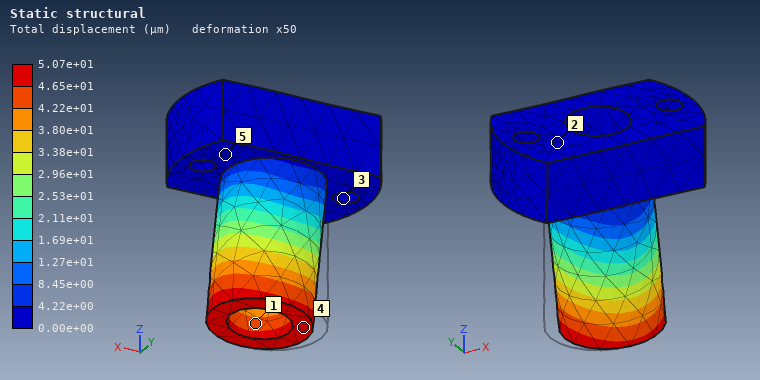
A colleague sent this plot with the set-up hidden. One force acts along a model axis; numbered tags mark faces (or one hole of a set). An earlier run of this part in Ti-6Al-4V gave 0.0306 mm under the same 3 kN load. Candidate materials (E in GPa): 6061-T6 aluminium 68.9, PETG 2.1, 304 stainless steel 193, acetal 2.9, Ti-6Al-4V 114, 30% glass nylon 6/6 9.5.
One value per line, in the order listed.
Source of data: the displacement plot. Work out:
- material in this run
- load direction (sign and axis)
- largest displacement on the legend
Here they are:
6061-T6 aluminium
+X
5.07e+01 µm
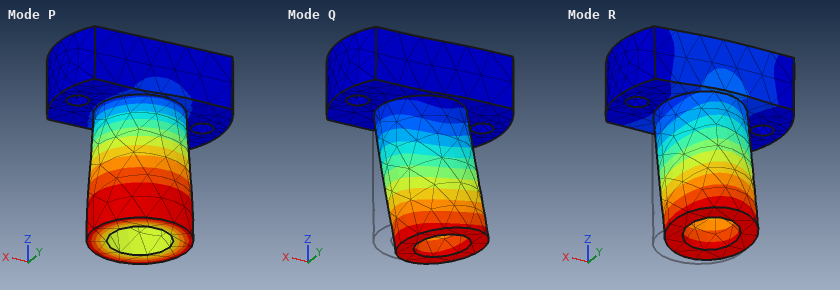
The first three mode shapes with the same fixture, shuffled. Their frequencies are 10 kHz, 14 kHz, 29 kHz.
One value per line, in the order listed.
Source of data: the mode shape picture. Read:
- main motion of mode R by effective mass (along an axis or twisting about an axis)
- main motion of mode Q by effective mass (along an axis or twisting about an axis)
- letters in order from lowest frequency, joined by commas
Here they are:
along Y
along X
R, Q, P
